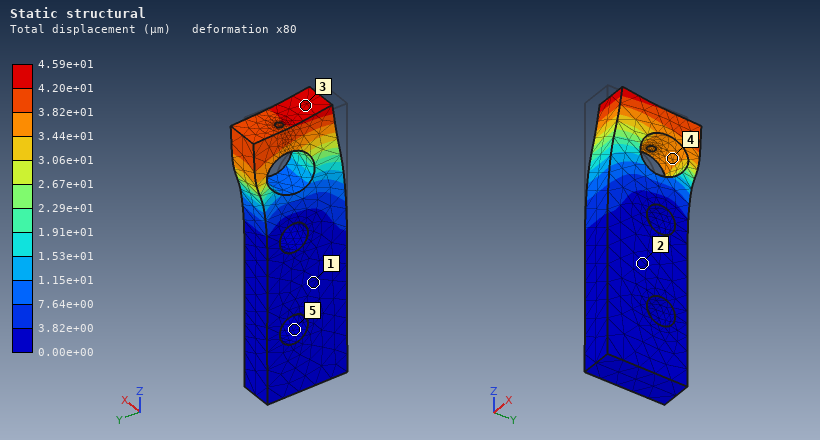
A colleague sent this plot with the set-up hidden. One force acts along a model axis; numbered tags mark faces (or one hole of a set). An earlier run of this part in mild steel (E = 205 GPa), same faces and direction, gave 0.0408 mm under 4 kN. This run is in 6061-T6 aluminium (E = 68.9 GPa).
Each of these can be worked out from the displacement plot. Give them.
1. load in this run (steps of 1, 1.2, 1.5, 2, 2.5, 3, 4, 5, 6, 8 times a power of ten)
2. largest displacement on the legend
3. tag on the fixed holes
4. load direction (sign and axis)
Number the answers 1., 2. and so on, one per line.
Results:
1. 1.5 kN
2. 4.59e+01 µm
3. 5
4. +Y
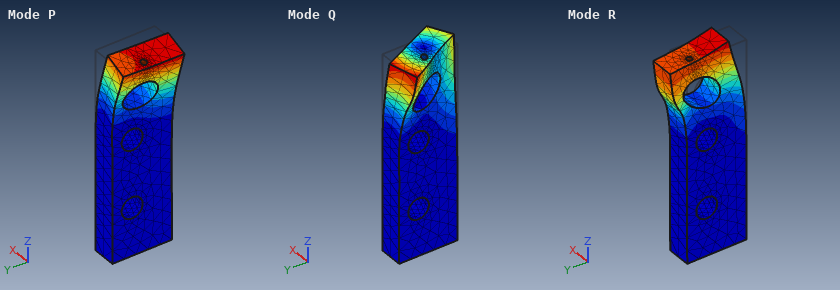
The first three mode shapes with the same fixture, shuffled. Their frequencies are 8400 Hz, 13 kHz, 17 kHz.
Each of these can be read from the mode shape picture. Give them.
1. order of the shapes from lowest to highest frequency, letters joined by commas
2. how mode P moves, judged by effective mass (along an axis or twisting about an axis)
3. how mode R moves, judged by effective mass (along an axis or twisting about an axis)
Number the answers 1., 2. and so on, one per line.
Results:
1. P, R, Q
2. along X
3. along Y
